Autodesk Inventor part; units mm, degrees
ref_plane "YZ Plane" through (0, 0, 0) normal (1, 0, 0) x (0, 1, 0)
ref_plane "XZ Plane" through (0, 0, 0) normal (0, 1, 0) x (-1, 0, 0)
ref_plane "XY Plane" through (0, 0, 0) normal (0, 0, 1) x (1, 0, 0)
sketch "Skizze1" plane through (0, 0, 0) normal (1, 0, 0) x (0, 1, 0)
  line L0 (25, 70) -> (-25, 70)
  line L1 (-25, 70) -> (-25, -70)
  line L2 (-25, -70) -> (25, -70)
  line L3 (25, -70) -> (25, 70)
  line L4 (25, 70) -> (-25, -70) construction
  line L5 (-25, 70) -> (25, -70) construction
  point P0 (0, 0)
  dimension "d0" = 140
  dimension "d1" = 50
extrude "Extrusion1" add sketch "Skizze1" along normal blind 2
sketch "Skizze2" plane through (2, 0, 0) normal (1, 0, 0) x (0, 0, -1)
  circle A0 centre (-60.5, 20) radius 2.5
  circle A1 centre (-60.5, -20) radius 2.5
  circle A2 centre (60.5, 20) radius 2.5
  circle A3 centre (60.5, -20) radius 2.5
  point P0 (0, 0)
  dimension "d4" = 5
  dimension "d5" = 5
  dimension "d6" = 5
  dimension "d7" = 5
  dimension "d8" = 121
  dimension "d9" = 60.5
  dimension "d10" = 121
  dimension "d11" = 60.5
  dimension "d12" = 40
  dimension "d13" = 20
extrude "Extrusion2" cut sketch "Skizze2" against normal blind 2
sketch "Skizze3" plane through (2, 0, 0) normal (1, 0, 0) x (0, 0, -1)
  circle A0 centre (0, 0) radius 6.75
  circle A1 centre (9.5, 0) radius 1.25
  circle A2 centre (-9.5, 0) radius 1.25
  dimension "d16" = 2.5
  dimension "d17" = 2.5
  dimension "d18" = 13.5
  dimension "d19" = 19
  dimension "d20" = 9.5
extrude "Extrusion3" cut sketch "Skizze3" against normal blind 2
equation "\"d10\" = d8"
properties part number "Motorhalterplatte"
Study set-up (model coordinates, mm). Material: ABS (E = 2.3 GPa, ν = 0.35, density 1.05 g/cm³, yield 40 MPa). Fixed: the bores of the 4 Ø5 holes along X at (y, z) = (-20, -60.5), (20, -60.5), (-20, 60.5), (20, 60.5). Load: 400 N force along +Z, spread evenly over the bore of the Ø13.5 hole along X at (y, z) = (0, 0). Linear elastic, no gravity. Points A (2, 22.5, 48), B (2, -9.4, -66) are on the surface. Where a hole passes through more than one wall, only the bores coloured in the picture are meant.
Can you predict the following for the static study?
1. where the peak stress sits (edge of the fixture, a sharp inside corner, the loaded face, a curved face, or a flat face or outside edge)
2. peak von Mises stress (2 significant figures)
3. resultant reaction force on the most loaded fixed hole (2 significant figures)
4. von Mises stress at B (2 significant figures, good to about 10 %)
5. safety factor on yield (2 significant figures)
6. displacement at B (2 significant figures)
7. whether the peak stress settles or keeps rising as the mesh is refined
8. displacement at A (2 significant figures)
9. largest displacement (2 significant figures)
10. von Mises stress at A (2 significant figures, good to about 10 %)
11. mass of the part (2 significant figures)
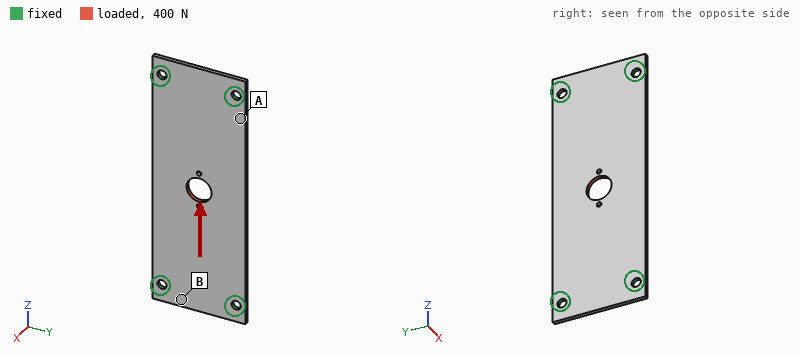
a curved face
16 MPa
100 N
0.95 MPa
2.5
17 µm
settles
17 µm
81 µm
2.9 MPa
14 g
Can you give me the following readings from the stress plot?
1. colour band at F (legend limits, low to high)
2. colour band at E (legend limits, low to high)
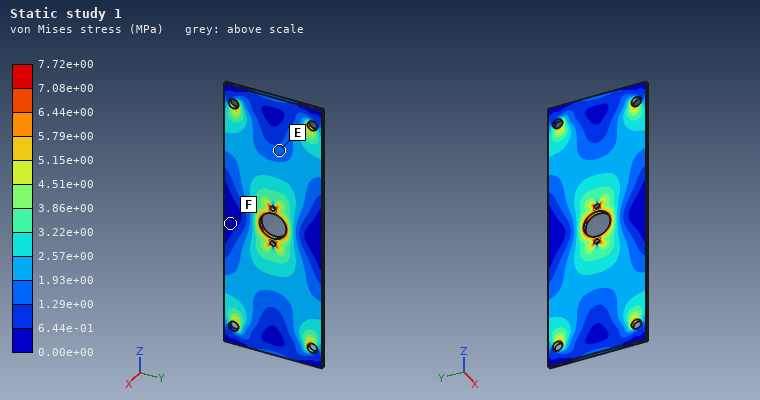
0.00e+00 to 6.44e-01 MPa
1.29e+00 to 1.93e+00 MPa
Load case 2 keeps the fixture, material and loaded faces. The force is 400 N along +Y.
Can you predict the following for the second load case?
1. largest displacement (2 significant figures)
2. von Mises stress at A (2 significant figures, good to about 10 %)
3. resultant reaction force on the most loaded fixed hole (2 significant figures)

0.24 mm
4.2 MPa
180 N
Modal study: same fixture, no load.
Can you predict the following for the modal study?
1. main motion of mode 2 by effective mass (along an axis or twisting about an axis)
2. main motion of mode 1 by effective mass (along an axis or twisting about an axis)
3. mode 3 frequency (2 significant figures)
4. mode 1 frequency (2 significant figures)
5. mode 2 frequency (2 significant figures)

twisting about Z
along X
570 Hz
210 Hz
400 Hz
